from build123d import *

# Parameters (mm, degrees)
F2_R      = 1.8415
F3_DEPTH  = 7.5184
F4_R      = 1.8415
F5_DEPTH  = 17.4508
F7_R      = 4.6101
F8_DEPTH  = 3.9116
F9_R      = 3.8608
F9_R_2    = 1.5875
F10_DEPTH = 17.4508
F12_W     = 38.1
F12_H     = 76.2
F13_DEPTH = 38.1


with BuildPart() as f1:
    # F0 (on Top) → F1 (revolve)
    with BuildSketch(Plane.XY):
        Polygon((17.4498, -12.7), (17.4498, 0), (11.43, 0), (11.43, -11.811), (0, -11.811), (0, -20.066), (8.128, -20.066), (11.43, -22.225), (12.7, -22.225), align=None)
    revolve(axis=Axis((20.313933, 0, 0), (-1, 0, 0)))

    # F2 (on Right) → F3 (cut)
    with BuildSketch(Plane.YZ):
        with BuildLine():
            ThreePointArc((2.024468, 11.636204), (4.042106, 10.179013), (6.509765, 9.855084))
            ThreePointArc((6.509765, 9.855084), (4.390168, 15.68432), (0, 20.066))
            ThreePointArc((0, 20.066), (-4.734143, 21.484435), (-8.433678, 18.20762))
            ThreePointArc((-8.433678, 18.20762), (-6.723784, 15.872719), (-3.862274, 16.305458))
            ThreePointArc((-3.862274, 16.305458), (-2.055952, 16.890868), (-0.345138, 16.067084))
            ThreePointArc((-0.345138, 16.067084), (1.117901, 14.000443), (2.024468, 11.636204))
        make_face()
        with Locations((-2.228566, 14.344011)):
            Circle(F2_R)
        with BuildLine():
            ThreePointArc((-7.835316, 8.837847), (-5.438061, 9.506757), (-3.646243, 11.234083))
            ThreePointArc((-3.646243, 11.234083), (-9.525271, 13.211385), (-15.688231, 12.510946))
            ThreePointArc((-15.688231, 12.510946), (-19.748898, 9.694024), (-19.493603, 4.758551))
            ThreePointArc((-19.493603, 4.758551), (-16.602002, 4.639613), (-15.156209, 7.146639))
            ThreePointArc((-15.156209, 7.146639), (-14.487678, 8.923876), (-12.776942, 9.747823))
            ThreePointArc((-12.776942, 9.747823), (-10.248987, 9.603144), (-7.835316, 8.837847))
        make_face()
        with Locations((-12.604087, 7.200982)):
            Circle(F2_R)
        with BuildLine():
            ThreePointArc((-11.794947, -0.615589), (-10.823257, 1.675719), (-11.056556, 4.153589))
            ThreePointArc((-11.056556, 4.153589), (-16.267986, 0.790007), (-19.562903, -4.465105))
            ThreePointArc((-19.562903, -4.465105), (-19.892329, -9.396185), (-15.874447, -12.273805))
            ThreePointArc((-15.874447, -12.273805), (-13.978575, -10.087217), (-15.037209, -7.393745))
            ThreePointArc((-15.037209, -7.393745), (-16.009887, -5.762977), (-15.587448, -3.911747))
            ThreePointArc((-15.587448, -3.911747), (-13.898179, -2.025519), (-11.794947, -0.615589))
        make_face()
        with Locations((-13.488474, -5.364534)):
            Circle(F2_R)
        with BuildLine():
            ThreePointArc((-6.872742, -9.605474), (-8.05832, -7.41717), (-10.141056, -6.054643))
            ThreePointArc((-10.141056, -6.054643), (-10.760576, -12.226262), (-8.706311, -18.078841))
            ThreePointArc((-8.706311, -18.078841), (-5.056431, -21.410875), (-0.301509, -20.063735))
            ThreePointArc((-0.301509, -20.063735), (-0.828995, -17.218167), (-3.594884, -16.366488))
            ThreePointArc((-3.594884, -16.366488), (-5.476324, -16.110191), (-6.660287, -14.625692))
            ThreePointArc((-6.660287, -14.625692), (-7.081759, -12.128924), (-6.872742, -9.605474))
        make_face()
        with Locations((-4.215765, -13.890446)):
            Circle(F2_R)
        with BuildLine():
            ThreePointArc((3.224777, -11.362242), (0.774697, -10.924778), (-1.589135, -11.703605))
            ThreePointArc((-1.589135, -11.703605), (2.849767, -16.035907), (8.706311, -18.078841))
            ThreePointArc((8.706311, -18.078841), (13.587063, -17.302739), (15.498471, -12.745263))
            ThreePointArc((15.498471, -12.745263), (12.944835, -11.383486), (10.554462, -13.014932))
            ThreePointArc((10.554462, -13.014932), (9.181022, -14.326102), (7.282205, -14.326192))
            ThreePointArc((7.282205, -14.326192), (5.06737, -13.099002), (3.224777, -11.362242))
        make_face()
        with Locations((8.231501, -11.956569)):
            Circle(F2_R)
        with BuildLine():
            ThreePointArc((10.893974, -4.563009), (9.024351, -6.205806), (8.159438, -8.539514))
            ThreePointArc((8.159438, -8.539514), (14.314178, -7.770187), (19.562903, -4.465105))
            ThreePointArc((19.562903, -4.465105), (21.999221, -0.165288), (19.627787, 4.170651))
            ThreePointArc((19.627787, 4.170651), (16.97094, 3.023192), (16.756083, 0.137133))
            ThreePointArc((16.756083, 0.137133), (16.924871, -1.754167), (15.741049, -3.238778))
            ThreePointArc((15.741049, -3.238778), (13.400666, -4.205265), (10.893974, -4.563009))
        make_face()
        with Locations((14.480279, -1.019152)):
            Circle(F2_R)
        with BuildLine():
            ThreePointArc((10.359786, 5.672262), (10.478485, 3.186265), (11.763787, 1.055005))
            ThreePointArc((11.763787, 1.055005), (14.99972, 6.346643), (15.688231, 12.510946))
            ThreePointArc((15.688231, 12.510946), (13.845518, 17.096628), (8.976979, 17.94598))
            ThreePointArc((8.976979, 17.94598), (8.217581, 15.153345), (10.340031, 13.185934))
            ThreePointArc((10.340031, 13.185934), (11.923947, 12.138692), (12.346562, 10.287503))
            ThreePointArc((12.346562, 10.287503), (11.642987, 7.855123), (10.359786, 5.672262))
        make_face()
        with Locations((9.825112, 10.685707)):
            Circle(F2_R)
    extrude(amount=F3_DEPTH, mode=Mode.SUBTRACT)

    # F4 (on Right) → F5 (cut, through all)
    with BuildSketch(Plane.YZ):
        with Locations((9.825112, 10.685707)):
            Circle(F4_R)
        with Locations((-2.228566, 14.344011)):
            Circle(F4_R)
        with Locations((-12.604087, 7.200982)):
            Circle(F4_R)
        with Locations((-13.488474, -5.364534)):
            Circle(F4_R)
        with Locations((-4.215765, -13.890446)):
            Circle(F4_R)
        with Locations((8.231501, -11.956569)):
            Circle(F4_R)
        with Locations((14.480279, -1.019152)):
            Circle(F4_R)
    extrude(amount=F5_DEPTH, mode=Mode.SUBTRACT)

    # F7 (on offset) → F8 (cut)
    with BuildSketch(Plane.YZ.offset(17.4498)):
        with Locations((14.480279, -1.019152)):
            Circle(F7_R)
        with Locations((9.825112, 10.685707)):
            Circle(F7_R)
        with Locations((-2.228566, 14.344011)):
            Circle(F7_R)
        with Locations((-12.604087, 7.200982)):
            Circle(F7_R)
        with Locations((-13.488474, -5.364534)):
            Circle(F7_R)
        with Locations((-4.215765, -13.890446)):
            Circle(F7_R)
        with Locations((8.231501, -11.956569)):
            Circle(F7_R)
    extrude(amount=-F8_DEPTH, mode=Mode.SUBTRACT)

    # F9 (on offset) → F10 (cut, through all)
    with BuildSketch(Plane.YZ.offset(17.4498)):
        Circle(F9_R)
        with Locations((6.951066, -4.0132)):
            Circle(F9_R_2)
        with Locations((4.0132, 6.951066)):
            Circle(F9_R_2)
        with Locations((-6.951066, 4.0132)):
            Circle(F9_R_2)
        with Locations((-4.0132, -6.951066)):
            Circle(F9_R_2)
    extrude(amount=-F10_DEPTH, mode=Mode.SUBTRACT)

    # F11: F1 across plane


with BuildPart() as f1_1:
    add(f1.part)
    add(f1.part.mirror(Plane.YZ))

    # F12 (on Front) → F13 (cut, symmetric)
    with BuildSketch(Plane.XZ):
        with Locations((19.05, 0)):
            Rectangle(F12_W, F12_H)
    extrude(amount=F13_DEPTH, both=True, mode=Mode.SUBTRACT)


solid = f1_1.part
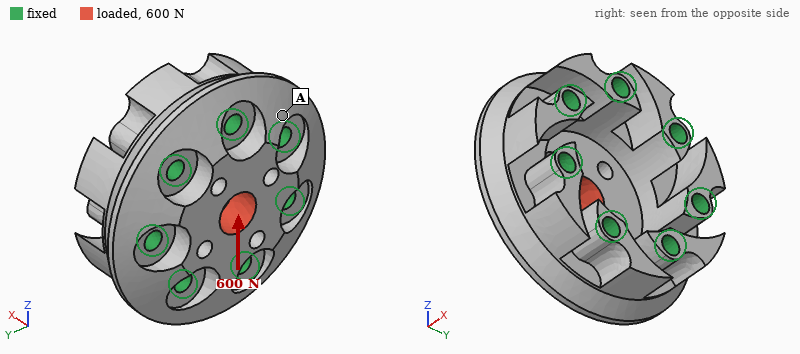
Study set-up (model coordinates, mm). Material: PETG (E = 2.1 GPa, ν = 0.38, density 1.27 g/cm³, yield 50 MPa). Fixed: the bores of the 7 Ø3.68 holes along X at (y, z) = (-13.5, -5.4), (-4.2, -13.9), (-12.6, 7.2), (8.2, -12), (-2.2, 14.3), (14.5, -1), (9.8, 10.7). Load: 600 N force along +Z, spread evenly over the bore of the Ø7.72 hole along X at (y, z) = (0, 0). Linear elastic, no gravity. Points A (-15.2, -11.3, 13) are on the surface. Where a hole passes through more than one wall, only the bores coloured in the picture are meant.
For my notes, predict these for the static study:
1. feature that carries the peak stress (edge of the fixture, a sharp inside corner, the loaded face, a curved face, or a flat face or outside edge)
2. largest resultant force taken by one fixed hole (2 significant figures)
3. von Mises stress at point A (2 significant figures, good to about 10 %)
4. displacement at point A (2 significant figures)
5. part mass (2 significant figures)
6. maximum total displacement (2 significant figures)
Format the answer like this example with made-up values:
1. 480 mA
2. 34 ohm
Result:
1. a curved face
2. 140 N
3. 1.4 MPa
4. 8.0 µm
5. 14 g
6. 35 µm
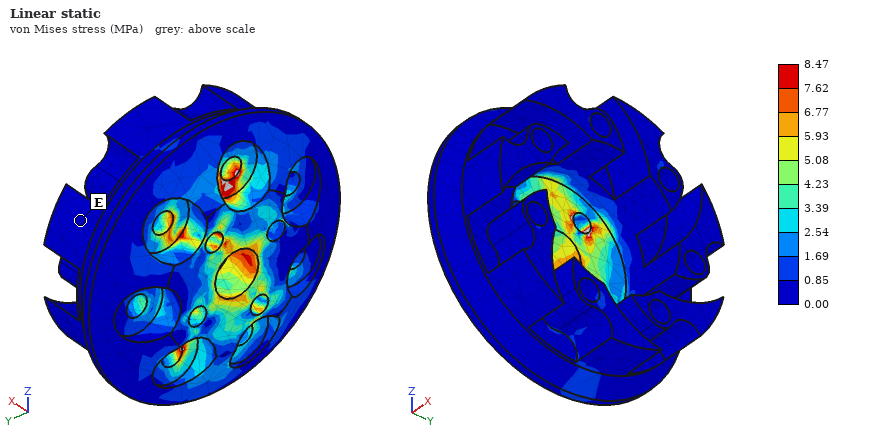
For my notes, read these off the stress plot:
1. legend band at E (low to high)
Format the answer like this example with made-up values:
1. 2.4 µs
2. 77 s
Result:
1. 0.00 to 0.85 MPa
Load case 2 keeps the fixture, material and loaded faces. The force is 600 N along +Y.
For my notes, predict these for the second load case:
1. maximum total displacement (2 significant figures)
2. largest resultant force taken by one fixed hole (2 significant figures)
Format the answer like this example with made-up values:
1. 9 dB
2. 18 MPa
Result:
1. 35 µm
2. 140 N
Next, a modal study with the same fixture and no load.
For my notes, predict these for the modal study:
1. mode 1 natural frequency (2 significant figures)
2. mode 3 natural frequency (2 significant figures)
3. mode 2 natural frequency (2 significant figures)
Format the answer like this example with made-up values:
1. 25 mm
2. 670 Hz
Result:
1. 12 kHz
2. 13 kHz
3. 13 kHz
